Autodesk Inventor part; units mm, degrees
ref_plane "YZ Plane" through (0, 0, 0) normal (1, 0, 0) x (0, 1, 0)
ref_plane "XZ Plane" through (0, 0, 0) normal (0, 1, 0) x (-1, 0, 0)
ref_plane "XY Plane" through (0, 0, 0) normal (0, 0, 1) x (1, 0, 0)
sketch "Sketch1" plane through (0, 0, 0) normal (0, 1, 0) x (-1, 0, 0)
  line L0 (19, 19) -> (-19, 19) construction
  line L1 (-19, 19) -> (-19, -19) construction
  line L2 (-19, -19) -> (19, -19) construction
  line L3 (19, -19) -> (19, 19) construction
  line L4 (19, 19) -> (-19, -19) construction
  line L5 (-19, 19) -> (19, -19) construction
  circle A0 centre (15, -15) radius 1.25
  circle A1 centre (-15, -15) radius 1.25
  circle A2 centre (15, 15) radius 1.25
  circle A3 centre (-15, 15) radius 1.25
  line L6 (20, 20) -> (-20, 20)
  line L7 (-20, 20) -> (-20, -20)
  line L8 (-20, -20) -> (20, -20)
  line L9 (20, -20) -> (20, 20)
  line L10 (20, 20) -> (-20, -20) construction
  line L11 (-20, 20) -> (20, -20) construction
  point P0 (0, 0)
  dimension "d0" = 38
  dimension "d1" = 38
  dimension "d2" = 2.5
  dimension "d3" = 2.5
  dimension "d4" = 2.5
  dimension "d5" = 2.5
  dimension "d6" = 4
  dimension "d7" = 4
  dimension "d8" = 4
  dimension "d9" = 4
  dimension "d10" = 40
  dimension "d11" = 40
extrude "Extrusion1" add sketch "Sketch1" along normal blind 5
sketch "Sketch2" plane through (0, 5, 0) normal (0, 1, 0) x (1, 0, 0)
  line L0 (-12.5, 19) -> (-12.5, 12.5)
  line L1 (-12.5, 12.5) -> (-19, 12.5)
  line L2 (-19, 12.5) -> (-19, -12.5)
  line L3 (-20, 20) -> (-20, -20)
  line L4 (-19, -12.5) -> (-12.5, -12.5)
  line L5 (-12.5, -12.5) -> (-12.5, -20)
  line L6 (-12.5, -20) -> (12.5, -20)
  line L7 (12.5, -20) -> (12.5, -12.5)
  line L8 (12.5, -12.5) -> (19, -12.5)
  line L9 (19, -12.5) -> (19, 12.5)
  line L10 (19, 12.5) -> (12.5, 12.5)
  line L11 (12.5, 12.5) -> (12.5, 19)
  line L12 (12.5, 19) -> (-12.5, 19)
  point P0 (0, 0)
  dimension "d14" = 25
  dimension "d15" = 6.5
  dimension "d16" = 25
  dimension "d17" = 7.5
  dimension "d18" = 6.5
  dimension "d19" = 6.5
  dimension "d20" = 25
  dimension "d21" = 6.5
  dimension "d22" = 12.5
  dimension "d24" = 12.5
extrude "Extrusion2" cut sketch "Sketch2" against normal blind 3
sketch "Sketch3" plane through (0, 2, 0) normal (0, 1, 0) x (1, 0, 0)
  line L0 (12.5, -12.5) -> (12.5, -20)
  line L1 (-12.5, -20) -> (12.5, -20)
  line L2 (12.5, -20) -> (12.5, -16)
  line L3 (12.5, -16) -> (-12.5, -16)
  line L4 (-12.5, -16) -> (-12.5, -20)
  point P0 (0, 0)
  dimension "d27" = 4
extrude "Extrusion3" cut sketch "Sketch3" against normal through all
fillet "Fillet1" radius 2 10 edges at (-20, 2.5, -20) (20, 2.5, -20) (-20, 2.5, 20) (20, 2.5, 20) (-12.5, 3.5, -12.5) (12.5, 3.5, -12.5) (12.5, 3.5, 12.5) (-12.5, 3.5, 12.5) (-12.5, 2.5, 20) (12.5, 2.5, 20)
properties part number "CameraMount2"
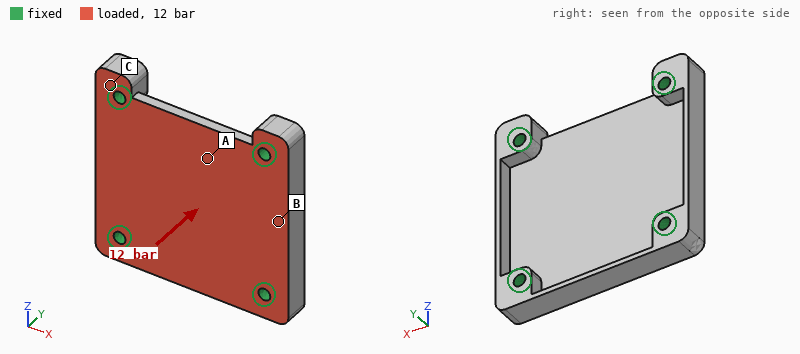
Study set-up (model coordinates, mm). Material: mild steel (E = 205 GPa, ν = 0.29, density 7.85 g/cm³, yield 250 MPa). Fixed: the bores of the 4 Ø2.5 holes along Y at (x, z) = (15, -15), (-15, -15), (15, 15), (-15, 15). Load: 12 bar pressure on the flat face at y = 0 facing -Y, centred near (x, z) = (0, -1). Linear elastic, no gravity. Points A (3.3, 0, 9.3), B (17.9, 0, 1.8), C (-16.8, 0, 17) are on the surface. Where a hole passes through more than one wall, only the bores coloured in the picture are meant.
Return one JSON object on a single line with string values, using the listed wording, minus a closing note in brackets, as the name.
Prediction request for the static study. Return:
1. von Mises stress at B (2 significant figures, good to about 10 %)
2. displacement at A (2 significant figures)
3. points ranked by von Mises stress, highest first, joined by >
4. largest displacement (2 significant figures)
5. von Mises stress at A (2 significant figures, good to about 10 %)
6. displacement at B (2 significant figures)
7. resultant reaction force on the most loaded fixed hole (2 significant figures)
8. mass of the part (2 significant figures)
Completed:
{"von Mises stress at B": "39 MPa", "displacement at A": "27 µm", "points ranked by von Mises stress, highest first, joined by >": "A > B > C", "largest displacement": "36 µm", "von Mises stress at A": "65 MPa", "displacement at B": "8.1 µm", "resultant reaction force on the most loaded fixed hole": "490 N", "mass of the part": "30 g"}
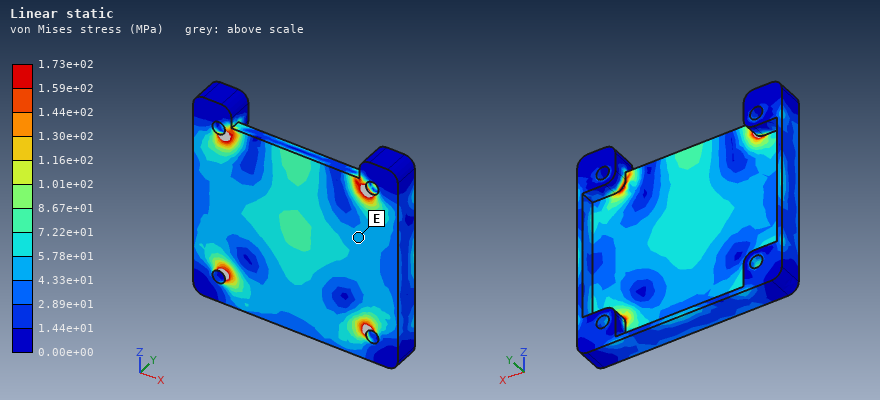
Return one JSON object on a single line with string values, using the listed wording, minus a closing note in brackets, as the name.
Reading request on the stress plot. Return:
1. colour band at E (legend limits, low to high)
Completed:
{"colour band at E": "4.33e+01 to 5.78e+01 MPa"}
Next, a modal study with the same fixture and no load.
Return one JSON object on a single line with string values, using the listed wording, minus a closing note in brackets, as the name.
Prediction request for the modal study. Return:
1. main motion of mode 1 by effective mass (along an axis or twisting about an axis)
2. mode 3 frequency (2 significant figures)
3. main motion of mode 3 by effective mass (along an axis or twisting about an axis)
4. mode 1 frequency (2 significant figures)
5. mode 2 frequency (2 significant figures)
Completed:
{"main motion of mode 1 by effective mass": "along Y", "mode 3 frequency": "18 kHz", "main motion of mode 3 by effective mass": "twisting about Z", "mode 1 frequency": "9100 Hz", "mode 2 frequency": "16 kHz"}
